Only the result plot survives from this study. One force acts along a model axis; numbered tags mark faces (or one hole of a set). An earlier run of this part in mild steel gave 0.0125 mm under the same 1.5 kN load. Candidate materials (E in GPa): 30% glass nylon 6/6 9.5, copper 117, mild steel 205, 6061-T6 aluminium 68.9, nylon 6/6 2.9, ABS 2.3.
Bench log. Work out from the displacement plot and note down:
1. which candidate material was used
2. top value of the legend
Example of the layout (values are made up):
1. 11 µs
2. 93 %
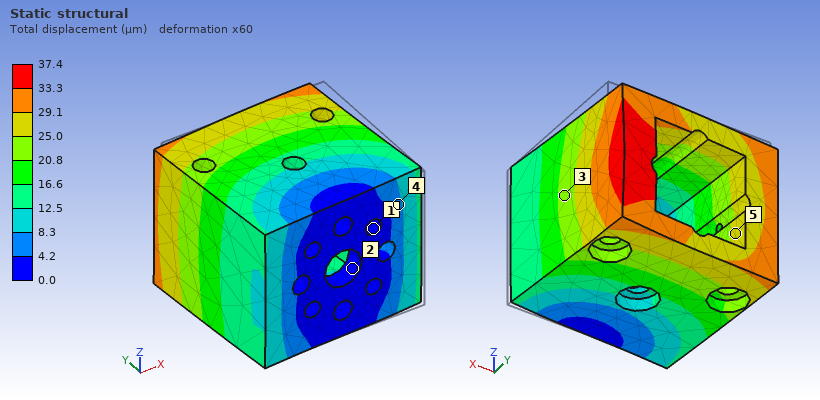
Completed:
1. 6061-T6 aluminium
2. 37.4 µm
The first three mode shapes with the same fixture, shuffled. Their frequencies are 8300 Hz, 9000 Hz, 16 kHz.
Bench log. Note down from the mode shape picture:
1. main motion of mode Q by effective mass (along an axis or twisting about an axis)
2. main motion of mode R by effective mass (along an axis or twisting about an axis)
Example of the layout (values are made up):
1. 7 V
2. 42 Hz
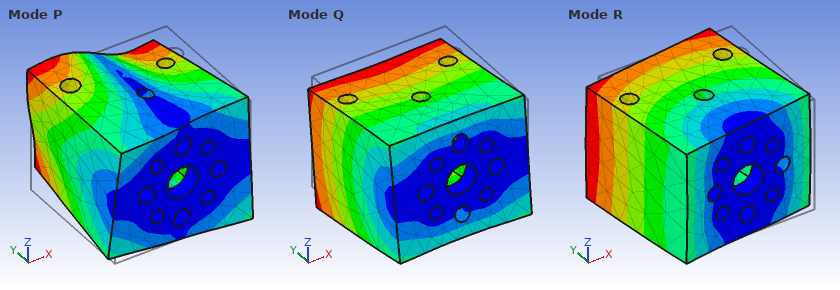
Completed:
1. along Z
2. along X
